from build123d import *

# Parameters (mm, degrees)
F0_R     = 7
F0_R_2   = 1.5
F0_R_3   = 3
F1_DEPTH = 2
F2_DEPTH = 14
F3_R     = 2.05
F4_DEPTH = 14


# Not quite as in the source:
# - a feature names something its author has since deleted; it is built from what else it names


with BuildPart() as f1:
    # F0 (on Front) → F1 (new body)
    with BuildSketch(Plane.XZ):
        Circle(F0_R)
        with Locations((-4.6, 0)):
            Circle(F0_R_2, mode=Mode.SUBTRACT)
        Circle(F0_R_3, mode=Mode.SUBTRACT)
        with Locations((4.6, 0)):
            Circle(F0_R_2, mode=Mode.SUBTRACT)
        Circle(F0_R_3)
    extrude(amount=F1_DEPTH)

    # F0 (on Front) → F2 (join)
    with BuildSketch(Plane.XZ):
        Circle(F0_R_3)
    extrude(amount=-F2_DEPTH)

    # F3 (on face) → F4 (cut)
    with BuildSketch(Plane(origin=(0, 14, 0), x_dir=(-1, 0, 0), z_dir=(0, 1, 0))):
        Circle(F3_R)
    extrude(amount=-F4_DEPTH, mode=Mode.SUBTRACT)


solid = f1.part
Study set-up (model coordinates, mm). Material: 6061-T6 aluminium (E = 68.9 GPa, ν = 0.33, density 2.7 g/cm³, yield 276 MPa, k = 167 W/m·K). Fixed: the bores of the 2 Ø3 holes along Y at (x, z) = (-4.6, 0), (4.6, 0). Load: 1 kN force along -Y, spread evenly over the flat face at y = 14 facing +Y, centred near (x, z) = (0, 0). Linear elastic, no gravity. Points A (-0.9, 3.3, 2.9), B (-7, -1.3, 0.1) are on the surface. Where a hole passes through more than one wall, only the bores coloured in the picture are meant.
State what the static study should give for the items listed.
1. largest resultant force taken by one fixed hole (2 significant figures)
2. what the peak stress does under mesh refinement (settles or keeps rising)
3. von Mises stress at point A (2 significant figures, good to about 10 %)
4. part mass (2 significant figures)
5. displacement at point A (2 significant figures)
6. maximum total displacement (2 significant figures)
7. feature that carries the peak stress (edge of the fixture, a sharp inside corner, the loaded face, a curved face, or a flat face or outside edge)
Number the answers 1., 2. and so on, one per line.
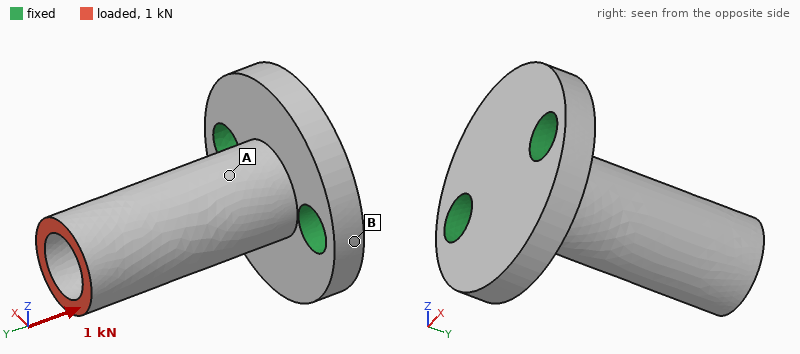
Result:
1. 510 N
2. keeps rising
3. 56 MPa
4. 1.3 g
5. 7.1 µm
6. 17 µm
7. edge of the fixture
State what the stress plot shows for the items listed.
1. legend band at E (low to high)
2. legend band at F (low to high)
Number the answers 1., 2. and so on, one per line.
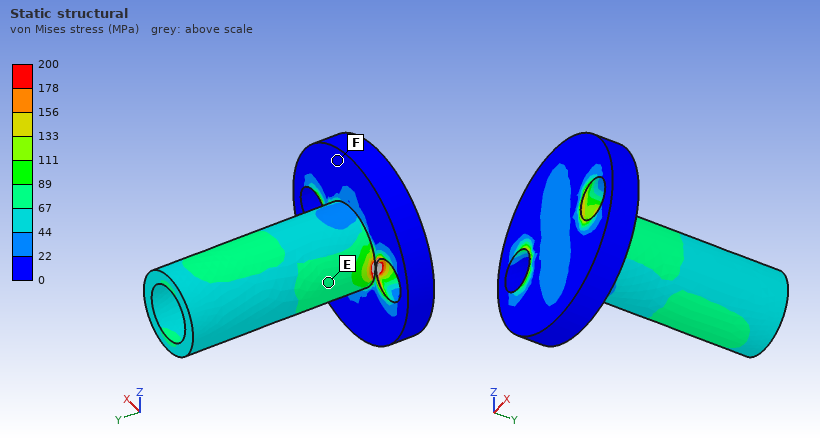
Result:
1. 67 to 89 MPa
2. 0 to 22 MPa
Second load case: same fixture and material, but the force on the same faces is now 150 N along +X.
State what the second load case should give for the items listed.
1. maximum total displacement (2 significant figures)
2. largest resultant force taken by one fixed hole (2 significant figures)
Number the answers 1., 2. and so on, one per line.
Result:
1. 62 µm
2. 350 N
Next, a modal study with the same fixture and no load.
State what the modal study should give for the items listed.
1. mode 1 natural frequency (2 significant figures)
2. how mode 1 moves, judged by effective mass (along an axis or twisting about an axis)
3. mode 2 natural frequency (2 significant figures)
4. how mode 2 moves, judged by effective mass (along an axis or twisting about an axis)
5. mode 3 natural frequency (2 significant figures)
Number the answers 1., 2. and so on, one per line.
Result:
1. 15 kHz
2. along Z
3. 20 kHz
4. along X
5. 53 kHz
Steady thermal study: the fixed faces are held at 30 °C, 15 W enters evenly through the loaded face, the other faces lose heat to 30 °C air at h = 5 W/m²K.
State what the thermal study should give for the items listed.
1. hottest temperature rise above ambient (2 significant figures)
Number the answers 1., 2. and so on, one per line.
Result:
1. 90 K
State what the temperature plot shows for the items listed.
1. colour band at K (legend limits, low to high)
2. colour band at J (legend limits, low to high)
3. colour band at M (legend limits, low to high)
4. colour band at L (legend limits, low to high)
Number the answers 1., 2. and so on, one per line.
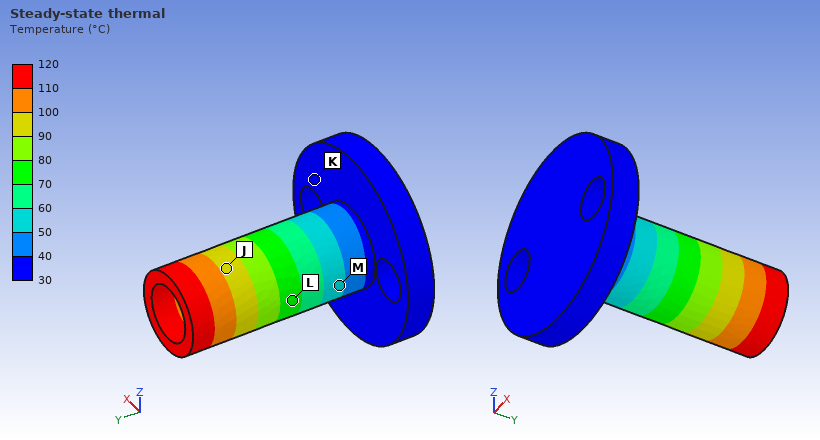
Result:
1. 30 to 40 °C
2. 90 to 100 °C
3. 50 to 60 °C
4. 70 to 80 °C
